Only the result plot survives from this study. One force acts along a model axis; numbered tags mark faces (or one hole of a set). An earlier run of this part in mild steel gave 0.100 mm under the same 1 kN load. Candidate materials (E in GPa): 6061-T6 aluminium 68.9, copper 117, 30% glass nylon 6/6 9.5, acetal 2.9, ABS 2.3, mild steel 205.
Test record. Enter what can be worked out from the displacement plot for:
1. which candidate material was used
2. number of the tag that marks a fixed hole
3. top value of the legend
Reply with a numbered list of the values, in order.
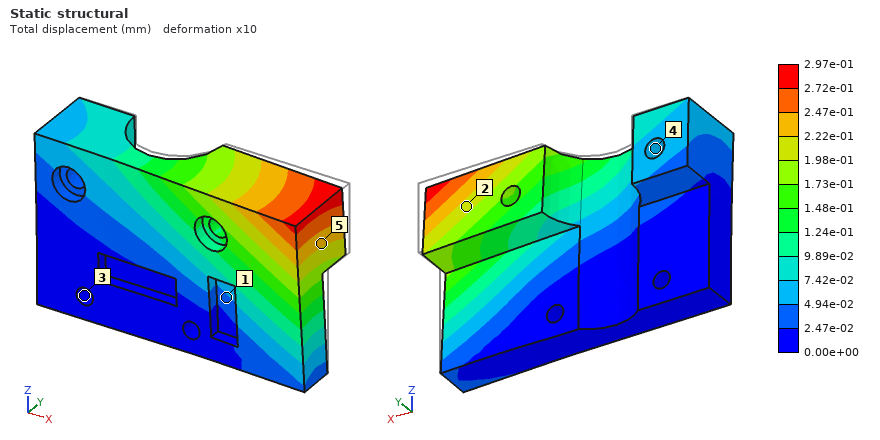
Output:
1. 6061-T6 aluminium
2. 3
3. 2.97e-01 mm
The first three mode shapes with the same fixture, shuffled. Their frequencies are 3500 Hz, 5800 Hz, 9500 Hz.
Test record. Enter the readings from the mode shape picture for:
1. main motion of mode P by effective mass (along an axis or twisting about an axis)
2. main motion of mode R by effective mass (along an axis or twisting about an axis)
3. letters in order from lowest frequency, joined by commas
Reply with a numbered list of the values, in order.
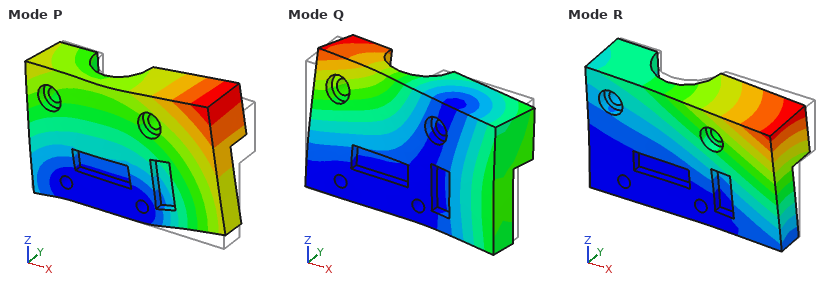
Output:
1. along X
2. along Y
3. R, Q, P
